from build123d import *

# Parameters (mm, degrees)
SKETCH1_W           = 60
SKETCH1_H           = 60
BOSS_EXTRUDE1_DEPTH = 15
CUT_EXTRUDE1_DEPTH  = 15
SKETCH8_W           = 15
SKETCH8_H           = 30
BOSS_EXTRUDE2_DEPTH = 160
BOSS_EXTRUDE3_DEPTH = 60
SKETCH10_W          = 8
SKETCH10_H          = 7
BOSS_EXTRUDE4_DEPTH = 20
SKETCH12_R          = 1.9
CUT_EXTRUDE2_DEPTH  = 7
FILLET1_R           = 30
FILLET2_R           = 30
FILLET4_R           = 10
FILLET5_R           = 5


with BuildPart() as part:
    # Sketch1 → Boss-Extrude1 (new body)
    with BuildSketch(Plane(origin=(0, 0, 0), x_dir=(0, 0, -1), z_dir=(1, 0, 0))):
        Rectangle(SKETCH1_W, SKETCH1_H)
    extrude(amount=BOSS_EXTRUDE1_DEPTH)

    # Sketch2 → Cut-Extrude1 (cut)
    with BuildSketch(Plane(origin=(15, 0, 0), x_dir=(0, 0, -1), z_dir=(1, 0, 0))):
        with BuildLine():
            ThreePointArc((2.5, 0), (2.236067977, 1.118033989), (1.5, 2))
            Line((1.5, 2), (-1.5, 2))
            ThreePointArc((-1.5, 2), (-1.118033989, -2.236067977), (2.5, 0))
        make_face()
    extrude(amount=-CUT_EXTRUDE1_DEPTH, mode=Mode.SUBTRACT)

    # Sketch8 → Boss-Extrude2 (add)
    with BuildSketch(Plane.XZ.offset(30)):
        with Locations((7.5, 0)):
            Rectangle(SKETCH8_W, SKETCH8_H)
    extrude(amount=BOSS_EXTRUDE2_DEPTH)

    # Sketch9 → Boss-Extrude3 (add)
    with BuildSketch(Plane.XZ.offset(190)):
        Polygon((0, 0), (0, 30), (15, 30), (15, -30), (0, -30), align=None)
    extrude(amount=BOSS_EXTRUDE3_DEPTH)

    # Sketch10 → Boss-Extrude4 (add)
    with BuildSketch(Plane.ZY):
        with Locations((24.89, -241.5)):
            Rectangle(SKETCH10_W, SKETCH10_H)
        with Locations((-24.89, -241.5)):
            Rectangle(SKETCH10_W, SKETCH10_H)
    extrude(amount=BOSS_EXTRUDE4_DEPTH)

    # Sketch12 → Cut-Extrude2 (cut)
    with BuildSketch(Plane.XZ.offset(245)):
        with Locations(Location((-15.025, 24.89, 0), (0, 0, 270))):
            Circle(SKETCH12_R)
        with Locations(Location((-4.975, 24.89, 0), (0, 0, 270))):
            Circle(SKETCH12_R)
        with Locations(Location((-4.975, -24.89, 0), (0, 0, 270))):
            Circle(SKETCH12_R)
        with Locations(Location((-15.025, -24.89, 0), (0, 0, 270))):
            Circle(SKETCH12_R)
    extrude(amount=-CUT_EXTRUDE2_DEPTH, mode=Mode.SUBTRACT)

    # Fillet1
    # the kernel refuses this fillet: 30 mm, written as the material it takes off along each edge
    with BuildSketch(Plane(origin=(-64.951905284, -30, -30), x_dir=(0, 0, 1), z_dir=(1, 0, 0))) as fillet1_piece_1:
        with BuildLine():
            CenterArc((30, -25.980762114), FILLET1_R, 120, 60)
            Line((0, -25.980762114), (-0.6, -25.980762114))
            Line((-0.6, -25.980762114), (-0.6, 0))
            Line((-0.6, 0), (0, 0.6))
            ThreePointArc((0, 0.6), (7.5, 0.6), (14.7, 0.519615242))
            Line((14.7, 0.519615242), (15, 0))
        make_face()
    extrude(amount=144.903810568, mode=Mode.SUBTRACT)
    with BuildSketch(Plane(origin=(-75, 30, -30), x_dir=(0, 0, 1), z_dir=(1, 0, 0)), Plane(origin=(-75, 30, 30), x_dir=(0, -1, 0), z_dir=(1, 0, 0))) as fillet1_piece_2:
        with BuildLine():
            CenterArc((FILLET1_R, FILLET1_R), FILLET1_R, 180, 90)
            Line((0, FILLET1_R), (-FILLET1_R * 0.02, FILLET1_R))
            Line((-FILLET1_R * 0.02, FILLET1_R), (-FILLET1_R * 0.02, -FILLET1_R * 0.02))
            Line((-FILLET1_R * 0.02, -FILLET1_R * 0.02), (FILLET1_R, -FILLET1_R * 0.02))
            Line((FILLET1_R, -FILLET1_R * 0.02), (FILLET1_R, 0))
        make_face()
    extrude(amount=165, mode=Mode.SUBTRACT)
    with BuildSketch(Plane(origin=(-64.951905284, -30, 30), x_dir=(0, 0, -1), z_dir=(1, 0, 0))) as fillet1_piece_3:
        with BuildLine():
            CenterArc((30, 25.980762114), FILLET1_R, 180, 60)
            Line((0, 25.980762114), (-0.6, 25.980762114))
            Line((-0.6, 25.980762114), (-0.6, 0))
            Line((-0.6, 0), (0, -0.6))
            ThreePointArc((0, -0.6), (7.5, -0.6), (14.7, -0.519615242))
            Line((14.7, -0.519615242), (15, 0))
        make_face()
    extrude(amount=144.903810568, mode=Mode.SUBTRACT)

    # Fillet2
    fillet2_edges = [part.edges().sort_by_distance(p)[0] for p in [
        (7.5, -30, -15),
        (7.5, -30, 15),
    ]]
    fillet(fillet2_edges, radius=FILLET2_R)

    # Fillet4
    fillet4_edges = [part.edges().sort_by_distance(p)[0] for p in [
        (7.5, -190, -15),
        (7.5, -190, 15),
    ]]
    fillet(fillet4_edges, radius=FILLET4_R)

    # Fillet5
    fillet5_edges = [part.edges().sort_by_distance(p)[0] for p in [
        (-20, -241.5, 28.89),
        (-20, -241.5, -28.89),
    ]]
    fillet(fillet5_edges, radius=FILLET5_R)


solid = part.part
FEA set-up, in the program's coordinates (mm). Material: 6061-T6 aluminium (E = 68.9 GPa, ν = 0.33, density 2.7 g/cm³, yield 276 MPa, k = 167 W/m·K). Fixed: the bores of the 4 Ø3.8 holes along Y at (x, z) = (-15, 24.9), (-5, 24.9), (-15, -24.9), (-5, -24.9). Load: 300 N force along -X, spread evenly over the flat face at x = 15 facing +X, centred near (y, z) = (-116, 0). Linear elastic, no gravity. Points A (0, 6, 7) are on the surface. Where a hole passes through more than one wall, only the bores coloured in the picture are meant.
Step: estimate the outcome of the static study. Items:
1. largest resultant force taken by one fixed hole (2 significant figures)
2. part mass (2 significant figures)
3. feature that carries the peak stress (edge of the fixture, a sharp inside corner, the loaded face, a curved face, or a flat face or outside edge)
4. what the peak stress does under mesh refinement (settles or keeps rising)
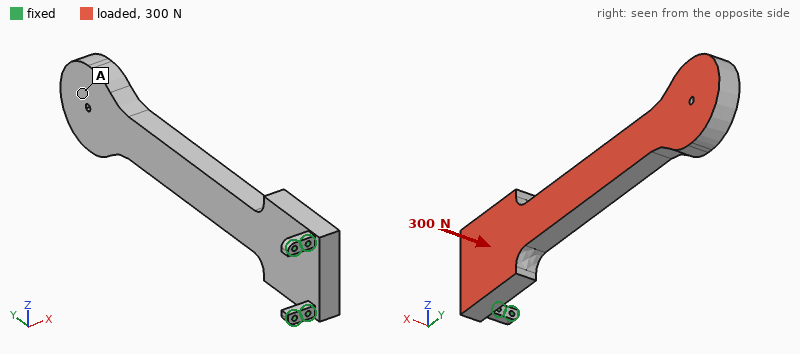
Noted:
200 N
470 g
edge of the fixture
keeps rising
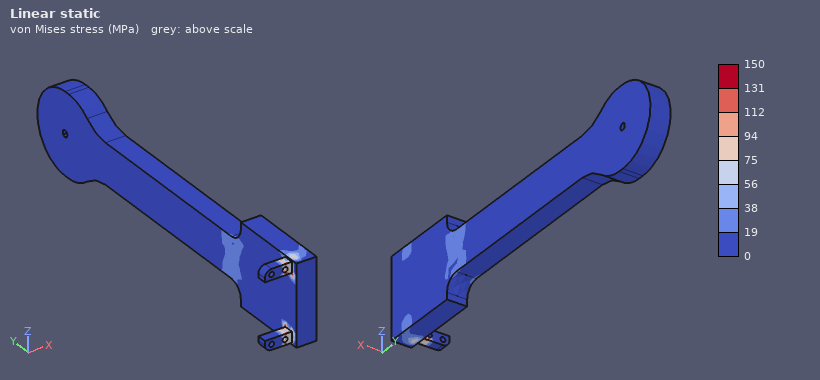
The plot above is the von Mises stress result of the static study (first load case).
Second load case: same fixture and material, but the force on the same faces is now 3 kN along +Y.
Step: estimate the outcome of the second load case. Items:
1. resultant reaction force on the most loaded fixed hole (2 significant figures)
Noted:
1.7 kN
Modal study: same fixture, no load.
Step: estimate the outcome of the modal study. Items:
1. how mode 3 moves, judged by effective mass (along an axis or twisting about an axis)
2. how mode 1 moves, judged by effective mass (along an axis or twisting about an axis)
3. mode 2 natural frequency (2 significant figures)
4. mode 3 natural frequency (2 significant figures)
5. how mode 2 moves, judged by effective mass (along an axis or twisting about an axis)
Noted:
along X
along X
330 Hz
740 Hz
along Z
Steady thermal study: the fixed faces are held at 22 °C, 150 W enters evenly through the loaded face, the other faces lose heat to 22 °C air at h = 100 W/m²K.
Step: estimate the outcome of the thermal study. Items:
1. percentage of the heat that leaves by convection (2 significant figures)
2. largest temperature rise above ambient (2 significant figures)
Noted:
64 %
60 K
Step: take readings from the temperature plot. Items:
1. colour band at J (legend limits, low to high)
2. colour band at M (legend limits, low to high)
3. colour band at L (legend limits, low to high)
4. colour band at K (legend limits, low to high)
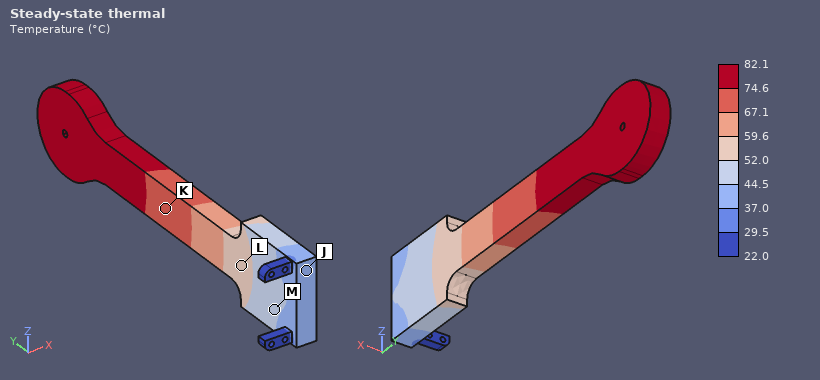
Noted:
37.0 to 44.5 °C
44.5 to 52.0 °C
52.0 to 59.6 °C
67.1 to 74.6 °C
